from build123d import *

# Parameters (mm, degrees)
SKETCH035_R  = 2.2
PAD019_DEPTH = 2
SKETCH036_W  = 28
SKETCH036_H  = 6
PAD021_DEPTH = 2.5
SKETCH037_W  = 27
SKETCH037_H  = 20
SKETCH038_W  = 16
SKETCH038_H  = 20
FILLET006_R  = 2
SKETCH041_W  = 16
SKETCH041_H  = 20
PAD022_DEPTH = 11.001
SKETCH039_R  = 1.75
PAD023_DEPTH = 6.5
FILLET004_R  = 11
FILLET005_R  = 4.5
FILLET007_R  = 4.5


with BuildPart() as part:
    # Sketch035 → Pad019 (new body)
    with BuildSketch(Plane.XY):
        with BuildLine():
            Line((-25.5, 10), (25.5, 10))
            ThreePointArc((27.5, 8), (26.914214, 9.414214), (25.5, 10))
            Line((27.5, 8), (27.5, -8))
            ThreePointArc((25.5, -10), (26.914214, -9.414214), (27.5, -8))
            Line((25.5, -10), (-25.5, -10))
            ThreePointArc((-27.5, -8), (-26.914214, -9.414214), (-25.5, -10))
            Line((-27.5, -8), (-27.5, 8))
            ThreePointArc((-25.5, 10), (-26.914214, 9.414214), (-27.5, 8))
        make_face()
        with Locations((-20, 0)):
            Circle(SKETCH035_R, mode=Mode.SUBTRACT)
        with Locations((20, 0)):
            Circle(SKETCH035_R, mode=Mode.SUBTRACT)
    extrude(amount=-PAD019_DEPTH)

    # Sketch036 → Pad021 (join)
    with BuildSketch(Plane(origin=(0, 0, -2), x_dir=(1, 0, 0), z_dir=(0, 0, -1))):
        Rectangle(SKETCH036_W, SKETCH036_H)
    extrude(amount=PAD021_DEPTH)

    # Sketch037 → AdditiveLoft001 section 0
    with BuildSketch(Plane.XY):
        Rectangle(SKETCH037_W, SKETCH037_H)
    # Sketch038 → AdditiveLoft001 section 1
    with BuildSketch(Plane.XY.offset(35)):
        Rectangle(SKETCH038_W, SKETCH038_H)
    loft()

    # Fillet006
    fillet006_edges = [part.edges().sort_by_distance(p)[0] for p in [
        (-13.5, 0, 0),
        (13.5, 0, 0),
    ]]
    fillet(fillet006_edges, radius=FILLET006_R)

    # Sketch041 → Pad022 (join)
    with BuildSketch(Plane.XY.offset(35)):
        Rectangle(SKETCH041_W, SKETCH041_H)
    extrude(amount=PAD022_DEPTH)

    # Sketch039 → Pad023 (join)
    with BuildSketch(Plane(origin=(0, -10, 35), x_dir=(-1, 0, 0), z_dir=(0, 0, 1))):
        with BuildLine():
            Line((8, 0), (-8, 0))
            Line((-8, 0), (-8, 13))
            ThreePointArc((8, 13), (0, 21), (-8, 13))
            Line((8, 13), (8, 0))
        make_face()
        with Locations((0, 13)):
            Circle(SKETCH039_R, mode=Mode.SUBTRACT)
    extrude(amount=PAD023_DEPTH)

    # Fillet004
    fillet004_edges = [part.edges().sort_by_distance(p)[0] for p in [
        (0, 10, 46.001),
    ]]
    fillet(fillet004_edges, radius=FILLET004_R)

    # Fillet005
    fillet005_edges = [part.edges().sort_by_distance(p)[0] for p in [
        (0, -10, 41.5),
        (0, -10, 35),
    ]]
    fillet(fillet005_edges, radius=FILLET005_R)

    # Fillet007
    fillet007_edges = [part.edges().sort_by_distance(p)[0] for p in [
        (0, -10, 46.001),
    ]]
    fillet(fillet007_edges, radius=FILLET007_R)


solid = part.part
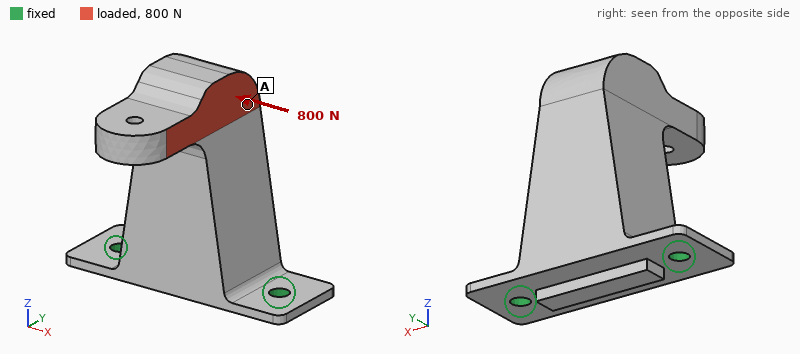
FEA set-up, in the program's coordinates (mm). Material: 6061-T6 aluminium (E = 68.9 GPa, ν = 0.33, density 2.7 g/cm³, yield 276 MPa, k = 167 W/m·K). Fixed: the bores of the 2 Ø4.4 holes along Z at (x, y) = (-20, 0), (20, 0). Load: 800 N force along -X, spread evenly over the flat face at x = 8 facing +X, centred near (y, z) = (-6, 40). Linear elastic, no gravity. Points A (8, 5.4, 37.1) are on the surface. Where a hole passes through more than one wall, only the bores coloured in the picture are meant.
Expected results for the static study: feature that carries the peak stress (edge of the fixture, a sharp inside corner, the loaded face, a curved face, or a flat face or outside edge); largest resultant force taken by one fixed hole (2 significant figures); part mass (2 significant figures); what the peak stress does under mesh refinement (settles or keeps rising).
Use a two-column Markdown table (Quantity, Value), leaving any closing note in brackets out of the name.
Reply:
| Quantity | Value |
|---|---|
| feature that carries the peak stress | edge of the fixture |
| largest resultant force taken by one fixed hole | 1.1 kN |
| part mass | 62 g |
| what the peak stress does under mesh refinement | keeps rising |
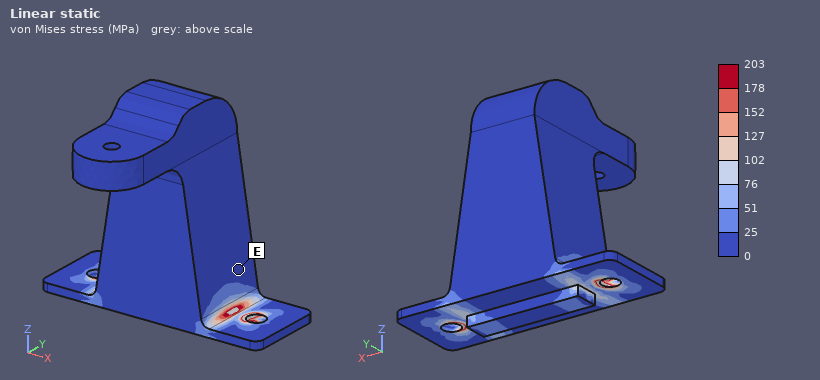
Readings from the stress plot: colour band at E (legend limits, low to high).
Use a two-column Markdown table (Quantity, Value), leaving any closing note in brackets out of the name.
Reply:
| Quantity | Value |
|---|---|
| colour band at E | 0 to 25 MPa |
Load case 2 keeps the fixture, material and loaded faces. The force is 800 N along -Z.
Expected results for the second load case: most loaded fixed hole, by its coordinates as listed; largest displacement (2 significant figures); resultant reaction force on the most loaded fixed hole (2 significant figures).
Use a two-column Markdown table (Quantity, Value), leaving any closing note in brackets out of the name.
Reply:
| Quantity | Value |
|---|---|
| most loaded fixed hole, by its coordinates as listed | (20, 0) |
| largest displacement | 0.30 mm |
| resultant reaction force on the most loaded fixed hole | 620 N |
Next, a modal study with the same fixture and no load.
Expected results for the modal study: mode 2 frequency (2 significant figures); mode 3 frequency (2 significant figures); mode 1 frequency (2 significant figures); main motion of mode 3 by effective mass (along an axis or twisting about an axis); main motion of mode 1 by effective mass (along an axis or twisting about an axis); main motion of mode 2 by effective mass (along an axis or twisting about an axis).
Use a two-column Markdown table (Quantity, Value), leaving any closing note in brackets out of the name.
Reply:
| Quantity | Value |
|---|---|
| mode 2 frequency | 3000 Hz |
| mode 3 frequency | 5000 Hz |
| mode 1 frequency | 710 Hz |
| main motion of mode 3 by effective mass | along Z |
| main motion of mode 1 by effective mass | along Y |
| main motion of mode 2 by effective mass | along X |
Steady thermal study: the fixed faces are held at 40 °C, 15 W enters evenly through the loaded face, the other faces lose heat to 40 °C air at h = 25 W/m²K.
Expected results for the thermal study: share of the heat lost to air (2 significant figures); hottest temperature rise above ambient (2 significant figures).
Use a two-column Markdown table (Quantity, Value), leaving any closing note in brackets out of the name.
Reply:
| Quantity | Value |
|---|---|
| share of the heat lost to air | 12 % |
| hottest temperature rise above ambient | 20 K |
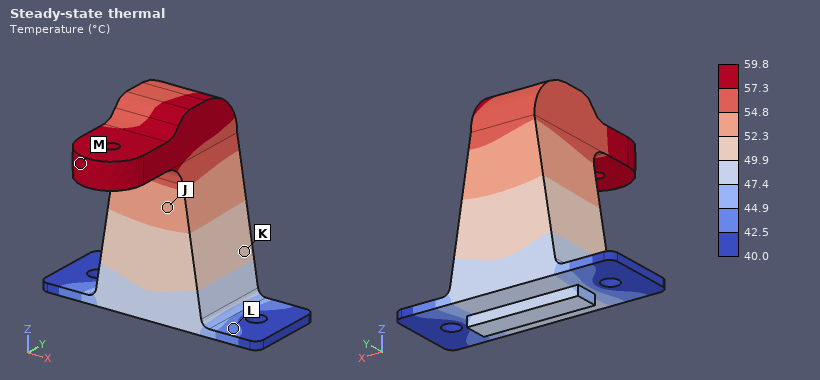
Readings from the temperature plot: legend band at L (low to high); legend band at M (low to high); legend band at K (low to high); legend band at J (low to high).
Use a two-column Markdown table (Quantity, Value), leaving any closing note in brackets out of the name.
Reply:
| Quantity | Value |
|---|---|
| legend band at L | 42.5 to 44.9 °C |
| legend band at M | 57.3 to 59.8 °C |
| legend band at K | 49.9 to 52.3 °C |
| legend band at J | 52.3 to 54.8 °C |
